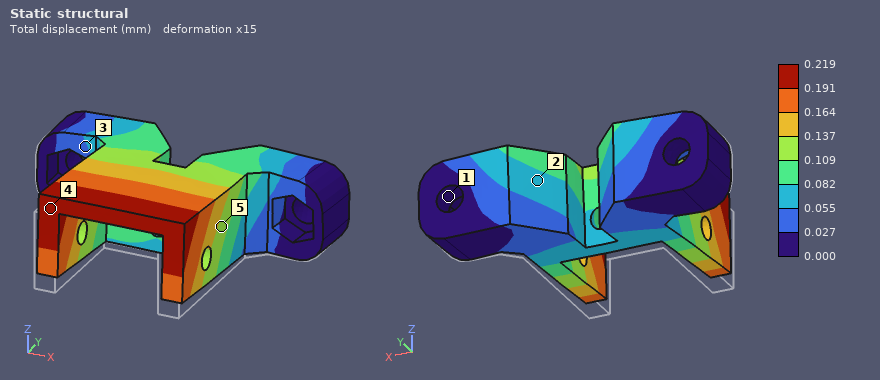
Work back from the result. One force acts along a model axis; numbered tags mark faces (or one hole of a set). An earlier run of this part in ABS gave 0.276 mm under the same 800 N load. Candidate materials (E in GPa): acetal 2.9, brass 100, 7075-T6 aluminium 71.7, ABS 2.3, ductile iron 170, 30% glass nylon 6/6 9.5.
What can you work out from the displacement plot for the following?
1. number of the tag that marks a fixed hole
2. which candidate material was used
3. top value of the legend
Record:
1
acetal
0.219 mm
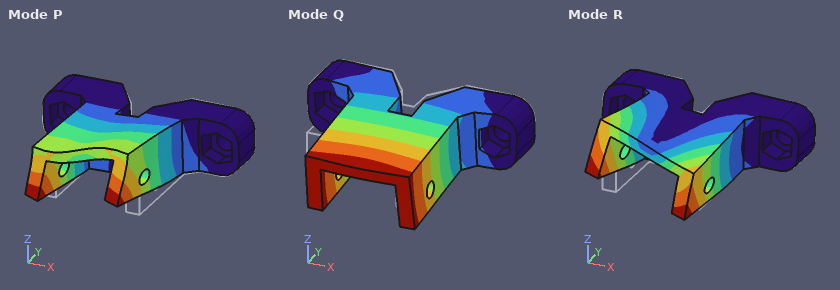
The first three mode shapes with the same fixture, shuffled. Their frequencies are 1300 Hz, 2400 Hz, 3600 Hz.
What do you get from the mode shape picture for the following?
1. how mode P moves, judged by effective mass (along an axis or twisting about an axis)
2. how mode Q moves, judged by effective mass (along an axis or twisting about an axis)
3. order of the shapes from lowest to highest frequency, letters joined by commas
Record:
along X
along Z
Q, R, P
